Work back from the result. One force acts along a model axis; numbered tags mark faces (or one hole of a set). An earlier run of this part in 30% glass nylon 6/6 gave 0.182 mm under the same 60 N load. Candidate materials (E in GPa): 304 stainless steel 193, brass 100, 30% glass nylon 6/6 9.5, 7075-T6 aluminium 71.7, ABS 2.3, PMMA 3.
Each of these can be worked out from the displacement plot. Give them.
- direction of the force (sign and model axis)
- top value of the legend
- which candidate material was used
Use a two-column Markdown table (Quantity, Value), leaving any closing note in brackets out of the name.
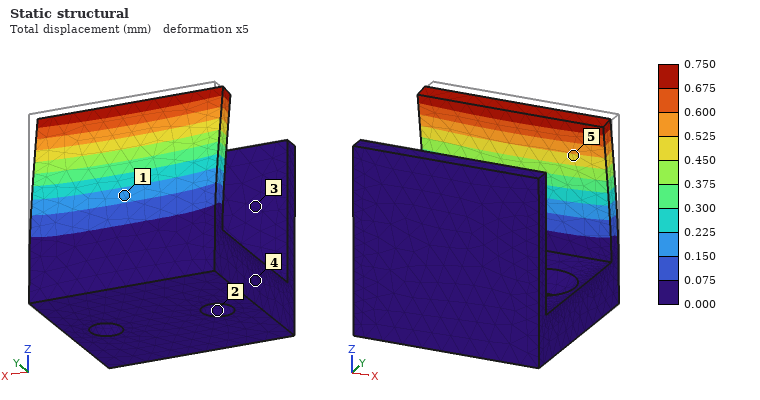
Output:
| Quantity | Value |
|---|---|
| direction of the force | -Y |
| top value of the legend | 0.750 mm |
| which candidate material was used | ABS |
